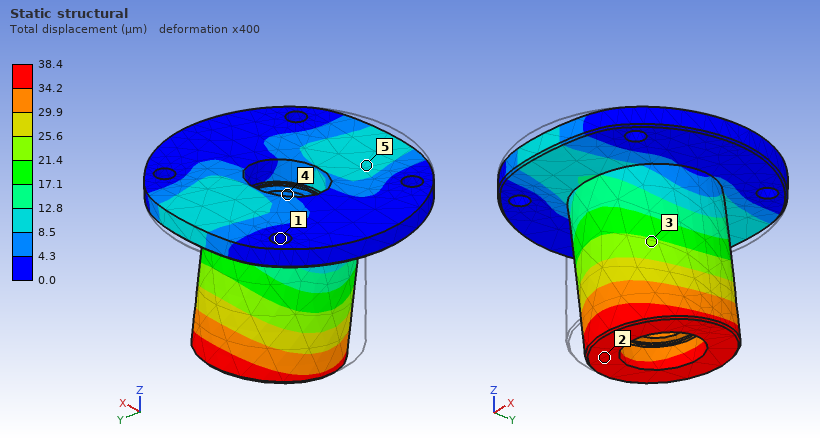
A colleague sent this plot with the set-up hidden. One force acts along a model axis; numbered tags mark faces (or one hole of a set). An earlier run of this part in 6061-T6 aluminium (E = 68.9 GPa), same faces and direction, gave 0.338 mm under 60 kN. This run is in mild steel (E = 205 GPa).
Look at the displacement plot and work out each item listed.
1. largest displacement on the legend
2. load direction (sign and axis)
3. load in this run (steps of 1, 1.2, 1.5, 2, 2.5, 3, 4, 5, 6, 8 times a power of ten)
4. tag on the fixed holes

38.4 µm
+Y
20 kN
1
